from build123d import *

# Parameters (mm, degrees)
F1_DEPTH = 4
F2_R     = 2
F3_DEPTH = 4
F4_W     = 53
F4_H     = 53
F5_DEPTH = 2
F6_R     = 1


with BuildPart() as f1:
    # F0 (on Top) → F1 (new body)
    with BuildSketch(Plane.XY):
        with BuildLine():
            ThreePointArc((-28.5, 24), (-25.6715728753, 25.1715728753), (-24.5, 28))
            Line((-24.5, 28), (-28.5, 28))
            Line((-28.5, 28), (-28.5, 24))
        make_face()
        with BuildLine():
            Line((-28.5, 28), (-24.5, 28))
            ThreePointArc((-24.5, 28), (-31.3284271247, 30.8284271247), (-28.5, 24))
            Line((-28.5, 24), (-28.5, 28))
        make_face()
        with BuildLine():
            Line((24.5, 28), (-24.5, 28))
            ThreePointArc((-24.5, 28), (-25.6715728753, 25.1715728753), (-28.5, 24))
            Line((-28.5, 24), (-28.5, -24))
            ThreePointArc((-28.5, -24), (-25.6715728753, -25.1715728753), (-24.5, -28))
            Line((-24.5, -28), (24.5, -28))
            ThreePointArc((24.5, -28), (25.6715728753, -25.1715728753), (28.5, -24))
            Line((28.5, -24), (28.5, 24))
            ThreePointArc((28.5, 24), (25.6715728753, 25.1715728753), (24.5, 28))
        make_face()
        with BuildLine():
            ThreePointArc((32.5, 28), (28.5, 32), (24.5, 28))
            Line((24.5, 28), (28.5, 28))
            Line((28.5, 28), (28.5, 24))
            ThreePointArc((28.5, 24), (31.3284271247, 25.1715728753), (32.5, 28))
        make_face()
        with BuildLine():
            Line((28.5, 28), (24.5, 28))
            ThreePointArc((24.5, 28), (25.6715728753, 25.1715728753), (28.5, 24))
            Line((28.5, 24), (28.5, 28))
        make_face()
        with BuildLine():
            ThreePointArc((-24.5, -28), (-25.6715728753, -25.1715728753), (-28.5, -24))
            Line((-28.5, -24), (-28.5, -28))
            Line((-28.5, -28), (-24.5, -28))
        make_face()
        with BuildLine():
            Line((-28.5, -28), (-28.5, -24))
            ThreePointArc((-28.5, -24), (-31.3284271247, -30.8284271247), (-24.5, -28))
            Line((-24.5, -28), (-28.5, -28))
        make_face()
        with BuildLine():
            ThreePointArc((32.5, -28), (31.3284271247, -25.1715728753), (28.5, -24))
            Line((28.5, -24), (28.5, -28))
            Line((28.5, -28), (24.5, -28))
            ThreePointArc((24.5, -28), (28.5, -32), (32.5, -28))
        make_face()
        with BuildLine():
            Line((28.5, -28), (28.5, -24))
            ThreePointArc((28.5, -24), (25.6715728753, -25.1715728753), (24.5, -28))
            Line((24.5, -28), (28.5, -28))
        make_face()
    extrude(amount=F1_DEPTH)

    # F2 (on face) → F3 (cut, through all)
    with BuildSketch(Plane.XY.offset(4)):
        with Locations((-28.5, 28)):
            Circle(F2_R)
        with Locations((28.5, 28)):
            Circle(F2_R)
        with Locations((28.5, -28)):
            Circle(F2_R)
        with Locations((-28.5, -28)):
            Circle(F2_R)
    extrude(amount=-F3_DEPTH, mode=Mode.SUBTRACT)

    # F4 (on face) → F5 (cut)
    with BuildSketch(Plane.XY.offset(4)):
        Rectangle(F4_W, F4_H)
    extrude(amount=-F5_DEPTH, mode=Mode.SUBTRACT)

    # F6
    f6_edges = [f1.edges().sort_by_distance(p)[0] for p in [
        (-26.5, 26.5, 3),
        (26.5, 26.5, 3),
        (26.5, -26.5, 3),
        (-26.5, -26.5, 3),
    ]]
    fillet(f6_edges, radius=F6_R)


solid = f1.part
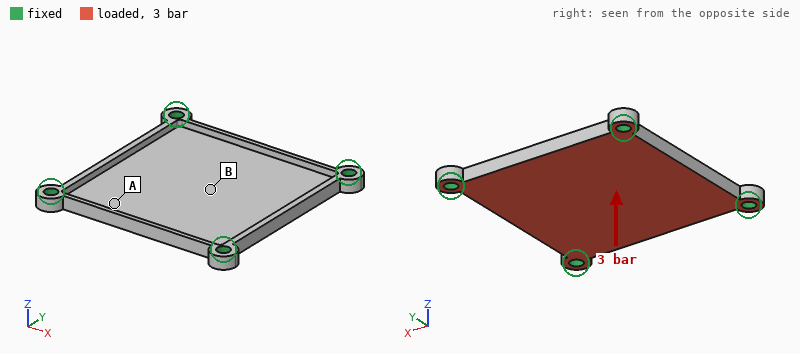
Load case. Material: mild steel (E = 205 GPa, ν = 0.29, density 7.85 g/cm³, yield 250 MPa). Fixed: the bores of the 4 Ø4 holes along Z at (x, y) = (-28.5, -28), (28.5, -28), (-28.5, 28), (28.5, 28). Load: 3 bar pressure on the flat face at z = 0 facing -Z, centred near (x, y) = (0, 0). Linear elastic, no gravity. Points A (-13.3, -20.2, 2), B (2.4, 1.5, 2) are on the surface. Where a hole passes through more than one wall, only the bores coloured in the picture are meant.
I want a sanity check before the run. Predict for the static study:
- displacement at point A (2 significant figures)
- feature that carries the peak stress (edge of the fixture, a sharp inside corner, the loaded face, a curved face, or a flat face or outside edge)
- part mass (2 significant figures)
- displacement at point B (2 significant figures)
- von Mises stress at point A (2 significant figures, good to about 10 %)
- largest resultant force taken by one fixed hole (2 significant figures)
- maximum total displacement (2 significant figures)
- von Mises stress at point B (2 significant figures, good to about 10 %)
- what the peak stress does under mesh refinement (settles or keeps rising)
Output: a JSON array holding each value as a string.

["40 µm", "a sharp inside corner", "59 g", "93 µm", "26 MPa", "350 N", "94 µm", "59 MPa", "keeps rising"]
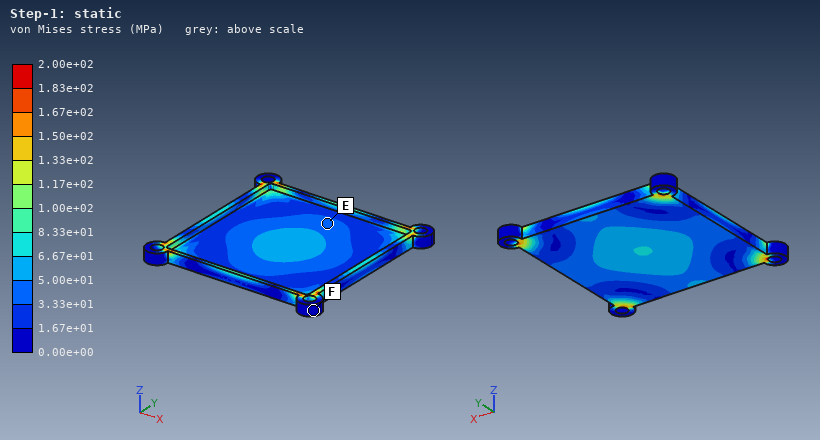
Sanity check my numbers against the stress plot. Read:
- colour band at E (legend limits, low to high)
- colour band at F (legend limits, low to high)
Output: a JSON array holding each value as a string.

["3.33e+01 to 5.00e+01 MPa", "0.00e+00 to 1.67e+01 MPa"]
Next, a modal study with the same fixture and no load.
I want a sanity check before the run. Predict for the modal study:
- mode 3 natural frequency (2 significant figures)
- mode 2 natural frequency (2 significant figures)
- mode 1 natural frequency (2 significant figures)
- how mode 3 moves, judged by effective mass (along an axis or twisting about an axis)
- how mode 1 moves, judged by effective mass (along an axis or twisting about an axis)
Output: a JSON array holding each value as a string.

["5400 Hz", "5200 Hz", "2800 Hz", "twisting about Y", "along Z"]
